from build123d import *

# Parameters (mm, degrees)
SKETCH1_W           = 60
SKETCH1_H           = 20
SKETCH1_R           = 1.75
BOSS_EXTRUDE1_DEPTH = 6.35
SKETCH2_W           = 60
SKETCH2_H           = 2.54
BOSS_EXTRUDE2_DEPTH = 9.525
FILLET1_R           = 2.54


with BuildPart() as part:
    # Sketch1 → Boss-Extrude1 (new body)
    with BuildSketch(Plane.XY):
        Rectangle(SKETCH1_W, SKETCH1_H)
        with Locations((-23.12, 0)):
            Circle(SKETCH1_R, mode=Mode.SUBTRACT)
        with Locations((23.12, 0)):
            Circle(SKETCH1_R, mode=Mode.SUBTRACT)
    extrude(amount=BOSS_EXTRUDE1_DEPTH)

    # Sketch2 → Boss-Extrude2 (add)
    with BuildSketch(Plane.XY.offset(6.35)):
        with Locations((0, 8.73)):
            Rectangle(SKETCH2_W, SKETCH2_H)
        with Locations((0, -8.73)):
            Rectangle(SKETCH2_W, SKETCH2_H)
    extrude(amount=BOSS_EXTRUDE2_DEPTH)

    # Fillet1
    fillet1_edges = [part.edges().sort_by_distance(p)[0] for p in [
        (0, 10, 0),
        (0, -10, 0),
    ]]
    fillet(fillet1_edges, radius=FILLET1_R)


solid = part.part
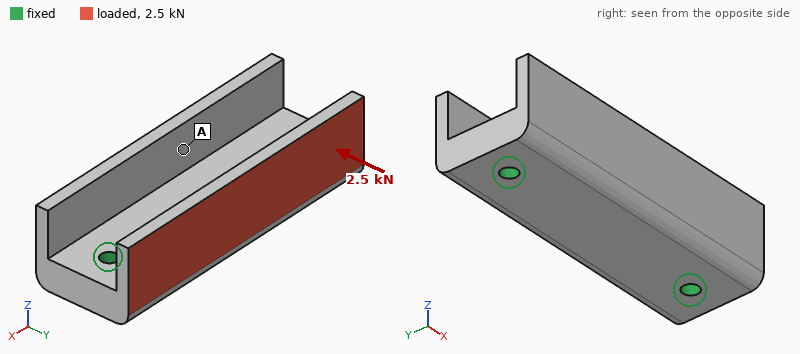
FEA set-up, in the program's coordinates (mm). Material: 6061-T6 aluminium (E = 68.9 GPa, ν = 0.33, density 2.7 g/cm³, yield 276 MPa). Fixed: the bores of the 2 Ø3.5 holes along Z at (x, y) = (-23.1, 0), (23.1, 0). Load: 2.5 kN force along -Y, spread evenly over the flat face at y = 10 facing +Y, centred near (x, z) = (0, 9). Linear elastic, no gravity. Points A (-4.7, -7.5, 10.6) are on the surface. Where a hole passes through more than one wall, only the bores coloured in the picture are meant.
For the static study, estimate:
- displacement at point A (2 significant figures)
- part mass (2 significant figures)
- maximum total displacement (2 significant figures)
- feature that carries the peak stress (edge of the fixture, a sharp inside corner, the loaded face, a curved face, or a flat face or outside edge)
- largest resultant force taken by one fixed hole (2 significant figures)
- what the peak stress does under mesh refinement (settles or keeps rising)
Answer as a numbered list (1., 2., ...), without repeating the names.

1. 23 µm
2. 28 g
3. 100 µm
4. edge of the fixture
5. 1.3 kN
6. keeps rising
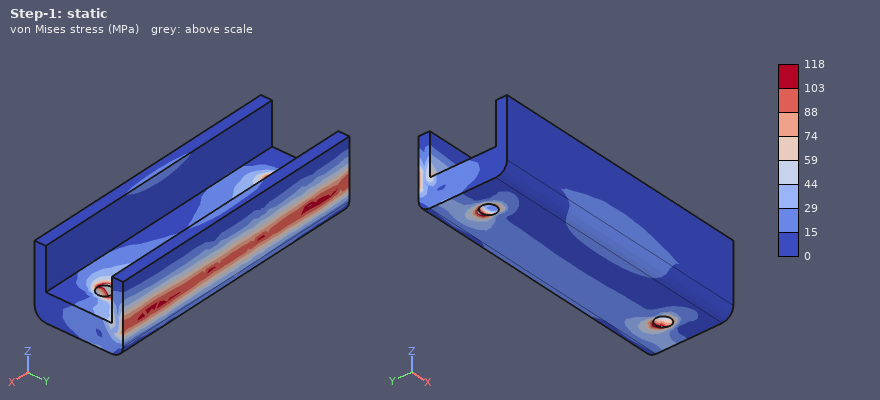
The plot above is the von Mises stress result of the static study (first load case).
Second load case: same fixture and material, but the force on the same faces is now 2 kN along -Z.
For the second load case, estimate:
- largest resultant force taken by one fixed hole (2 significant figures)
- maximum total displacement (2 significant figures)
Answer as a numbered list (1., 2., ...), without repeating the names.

1. 1.0 kN
2. 60 µm
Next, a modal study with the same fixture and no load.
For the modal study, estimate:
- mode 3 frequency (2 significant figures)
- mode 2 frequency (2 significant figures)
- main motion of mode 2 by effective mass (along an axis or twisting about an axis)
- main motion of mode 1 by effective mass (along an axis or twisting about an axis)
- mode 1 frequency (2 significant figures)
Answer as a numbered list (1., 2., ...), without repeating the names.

1. 16 kHz
2. 14 kHz
3. along Z
4. along Y
5. 11 kHz
